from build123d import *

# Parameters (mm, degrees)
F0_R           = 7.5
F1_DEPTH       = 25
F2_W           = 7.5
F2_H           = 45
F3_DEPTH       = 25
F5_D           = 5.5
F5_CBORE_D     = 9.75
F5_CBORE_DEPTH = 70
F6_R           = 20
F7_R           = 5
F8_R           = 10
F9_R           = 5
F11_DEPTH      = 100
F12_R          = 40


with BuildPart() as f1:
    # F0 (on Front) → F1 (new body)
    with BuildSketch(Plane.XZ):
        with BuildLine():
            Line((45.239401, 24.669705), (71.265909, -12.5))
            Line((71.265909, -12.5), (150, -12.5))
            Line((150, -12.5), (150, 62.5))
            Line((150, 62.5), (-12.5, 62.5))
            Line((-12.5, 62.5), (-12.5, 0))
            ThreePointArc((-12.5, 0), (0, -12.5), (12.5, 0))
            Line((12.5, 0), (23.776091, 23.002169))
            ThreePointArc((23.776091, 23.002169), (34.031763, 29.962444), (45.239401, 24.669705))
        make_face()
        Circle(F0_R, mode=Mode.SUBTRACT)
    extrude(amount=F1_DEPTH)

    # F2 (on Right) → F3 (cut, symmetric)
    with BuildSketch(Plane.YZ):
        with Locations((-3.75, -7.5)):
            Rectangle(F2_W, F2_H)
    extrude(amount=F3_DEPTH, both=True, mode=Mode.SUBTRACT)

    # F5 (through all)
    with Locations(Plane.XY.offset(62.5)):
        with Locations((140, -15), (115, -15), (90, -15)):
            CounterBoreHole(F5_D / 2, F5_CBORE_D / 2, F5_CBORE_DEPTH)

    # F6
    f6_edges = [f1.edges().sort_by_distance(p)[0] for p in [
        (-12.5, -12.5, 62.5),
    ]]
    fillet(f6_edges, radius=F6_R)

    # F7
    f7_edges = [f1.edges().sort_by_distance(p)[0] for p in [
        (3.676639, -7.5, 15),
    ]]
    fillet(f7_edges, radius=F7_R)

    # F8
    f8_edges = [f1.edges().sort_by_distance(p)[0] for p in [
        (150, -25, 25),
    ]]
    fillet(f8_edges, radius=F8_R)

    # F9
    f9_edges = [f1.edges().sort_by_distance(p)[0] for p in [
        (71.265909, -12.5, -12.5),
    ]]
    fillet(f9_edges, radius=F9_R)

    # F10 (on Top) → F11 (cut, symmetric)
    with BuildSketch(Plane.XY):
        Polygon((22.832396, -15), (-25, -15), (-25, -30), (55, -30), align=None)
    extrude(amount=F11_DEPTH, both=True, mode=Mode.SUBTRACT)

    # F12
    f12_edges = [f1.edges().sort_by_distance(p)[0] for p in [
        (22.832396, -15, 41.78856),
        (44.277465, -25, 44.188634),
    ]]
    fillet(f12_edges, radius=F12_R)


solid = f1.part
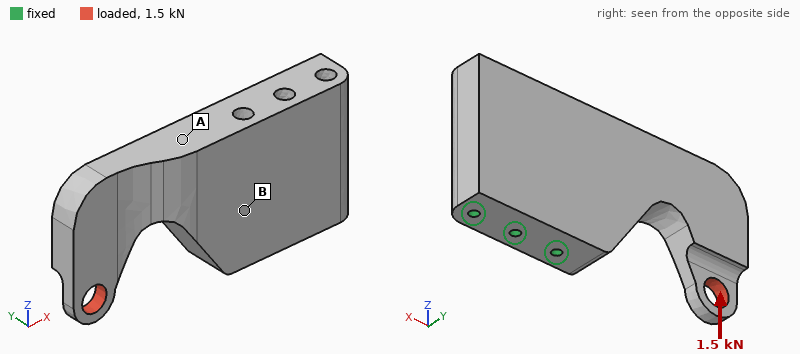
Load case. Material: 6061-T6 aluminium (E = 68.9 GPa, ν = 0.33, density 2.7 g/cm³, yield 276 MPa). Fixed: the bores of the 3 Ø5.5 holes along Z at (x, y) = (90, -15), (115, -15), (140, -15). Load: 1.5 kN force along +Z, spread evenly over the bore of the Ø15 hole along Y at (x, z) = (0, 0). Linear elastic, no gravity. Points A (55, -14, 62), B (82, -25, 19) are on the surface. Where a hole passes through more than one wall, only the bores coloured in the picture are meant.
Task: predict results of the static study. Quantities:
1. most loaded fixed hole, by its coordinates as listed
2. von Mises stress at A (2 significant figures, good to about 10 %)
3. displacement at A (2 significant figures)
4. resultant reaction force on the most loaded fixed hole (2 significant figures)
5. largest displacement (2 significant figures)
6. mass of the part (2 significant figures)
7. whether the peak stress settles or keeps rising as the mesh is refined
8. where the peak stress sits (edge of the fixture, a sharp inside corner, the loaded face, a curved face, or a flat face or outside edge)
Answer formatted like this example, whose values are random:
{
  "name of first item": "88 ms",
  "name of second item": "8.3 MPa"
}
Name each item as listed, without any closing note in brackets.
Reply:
{
  "most loaded fixed hole, by its coordinates as listed": "(90, -15)",
  "von Mises stress at A": "12 MPa",
  "displacement at A": "0.046 mm",
  "resultant reaction force on the most loaded fixed hole": "4.0 kN",
  "largest displacement": "0.11 mm",
  "mass of the part": "570 g",
  "whether the peak stress settles or keeps rising as the mesh is refined": "keeps rising",
  "where the peak stress sits": "edge of the fixture"
}
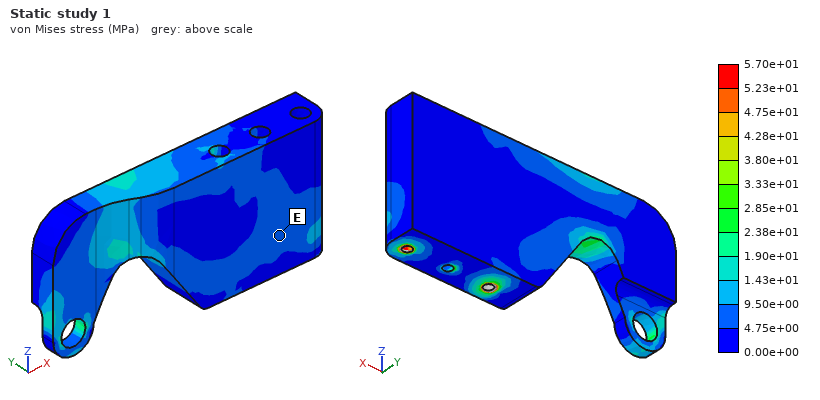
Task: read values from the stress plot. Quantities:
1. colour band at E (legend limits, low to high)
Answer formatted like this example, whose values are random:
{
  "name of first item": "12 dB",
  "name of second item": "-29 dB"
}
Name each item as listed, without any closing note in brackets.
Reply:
{
  "colour band at E": "4.75e+00 to 9.50e+00 MPa"
}
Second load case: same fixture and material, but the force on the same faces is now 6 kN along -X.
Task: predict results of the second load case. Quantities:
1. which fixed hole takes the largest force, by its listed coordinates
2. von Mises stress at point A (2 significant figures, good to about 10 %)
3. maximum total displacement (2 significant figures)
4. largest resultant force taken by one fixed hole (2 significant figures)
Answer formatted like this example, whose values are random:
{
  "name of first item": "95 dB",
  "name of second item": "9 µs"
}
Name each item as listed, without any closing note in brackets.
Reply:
{
  "which fixed hole takes the largest force, by its listed coordinates": "(90, -15)",
  "von Mises stress at point A": "34 MPa",
  "maximum total displacement": "0.35 mm",
  "largest resultant force taken by one fixed hole": "3.2 kN"
}
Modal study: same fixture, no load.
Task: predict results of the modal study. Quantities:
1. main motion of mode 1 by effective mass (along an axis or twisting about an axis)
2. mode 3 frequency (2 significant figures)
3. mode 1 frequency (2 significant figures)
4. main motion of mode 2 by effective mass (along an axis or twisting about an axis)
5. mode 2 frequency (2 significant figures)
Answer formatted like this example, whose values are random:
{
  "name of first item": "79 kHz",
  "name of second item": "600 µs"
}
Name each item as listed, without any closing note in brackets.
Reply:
{
  "main motion of mode 1 by effective mass": "along Y",
  "mode 3 frequency": "2000 Hz",
  "mode 1 frequency": "730 Hz",
  "main motion of mode 2 by effective mass": "twisting about Z",
  "mode 2 frequency": "1700 Hz"
}
